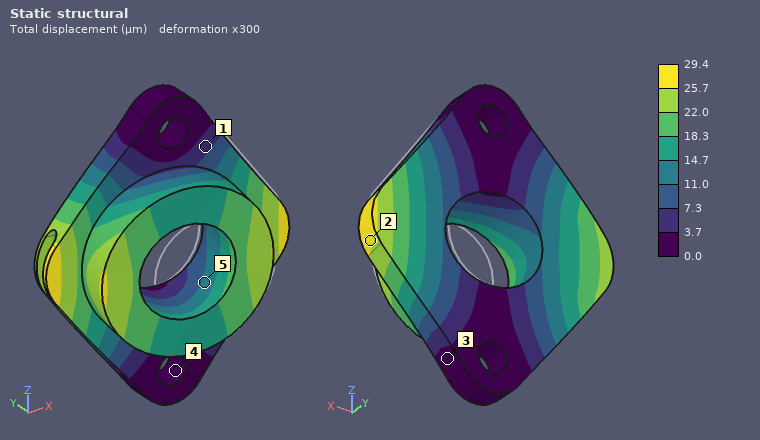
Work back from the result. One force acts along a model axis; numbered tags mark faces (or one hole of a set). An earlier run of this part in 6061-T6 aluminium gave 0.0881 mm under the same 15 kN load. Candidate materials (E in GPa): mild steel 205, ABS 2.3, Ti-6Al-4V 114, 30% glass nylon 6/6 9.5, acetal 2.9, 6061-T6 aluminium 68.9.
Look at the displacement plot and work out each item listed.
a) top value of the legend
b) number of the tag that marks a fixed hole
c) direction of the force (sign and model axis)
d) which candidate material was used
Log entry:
29.4 µm
4
-X
mild steel
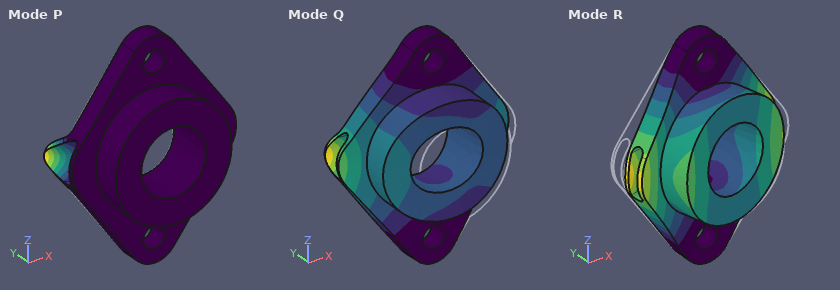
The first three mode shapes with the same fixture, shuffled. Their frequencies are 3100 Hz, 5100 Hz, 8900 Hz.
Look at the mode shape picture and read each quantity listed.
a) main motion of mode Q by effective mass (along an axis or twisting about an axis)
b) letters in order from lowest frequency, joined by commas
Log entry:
along Y
R, Q, P
